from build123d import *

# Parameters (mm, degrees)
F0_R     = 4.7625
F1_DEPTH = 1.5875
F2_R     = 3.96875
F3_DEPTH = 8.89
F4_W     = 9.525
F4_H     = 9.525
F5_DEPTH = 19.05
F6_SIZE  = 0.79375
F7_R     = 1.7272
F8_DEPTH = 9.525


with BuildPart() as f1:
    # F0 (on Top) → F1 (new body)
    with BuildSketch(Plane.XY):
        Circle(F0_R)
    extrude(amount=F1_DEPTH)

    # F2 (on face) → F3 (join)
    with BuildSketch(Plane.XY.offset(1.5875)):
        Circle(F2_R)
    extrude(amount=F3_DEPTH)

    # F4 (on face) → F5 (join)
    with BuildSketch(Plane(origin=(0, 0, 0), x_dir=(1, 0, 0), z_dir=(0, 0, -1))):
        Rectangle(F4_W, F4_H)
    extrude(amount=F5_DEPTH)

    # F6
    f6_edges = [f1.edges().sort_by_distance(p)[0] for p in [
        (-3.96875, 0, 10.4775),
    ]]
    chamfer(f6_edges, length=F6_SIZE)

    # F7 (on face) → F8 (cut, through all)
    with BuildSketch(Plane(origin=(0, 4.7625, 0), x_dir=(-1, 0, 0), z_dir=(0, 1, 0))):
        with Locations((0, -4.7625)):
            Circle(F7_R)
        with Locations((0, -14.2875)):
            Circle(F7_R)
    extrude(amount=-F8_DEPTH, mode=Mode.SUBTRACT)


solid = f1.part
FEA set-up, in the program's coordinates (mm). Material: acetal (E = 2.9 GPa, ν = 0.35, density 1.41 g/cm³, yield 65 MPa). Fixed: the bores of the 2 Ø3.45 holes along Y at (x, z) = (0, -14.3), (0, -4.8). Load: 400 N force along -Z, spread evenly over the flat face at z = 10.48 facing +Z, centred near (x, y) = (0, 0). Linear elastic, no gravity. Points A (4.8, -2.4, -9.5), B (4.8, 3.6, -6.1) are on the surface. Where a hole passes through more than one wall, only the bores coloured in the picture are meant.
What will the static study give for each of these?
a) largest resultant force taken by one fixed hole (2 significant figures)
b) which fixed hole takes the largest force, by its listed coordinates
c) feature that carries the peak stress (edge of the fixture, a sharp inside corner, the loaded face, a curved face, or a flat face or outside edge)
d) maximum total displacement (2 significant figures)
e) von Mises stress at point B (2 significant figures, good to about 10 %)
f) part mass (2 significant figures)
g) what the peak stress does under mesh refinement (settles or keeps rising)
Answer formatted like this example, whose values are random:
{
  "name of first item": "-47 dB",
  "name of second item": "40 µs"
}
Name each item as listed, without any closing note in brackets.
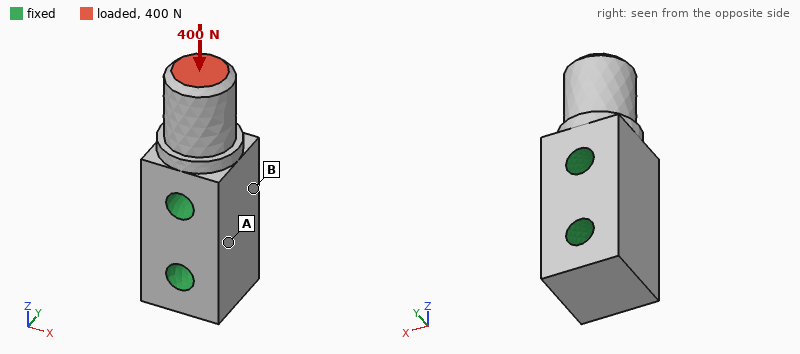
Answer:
{
  "largest resultant force taken by one fixed hole": "360 N",
  "which fixed hole takes the largest force, by its listed coordinates": "(0, -4.8)",
  "feature that carries the peak stress": "edge of the fixture",
  "maximum total displacement": "41 µm",
  "von Mises stress at point B": "2.0 MPa",
  "part mass": "3.0 g",
  "what the peak stress does under mesh refinement": "keeps rising"
}
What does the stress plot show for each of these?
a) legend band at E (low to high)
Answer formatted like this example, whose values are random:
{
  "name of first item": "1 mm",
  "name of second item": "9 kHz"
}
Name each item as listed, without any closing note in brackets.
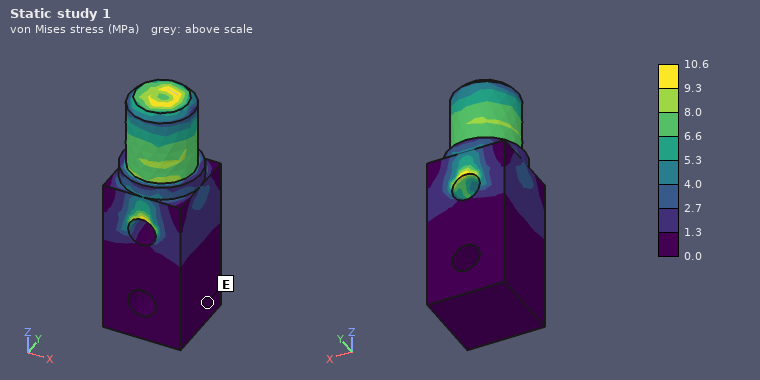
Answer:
{
  "legend band at E": "0.0 to 1.3 MPa"
}
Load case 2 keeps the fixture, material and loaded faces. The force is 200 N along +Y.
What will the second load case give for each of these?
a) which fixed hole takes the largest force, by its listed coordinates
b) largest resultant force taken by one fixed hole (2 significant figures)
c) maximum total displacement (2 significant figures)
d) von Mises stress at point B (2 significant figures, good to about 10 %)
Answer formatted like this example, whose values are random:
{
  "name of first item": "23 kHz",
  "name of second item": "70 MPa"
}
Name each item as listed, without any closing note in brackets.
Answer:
{
  "which fixed hole takes the largest force, by its listed coordinates": "(0, -4.8)",
  "largest resultant force taken by one fixed hole": "230 N",
  "maximum total displacement": "0.26 mm",
  "von Mises stress at point B": "5.8 MPa"
}
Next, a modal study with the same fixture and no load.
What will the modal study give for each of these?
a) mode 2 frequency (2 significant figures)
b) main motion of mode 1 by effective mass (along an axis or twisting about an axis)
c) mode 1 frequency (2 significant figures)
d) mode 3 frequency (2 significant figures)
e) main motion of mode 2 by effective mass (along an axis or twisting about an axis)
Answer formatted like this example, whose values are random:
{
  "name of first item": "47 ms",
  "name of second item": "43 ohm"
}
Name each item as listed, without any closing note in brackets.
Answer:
{
  "mode 2 frequency": "9300 Hz",
  "main motion of mode 1 by effective mass": "along X",
  "mode 1 frequency": "8000 Hz",
  "mode 3 frequency": "19 kHz",
  "main motion of mode 2 by effective mass": "along Y"
}
